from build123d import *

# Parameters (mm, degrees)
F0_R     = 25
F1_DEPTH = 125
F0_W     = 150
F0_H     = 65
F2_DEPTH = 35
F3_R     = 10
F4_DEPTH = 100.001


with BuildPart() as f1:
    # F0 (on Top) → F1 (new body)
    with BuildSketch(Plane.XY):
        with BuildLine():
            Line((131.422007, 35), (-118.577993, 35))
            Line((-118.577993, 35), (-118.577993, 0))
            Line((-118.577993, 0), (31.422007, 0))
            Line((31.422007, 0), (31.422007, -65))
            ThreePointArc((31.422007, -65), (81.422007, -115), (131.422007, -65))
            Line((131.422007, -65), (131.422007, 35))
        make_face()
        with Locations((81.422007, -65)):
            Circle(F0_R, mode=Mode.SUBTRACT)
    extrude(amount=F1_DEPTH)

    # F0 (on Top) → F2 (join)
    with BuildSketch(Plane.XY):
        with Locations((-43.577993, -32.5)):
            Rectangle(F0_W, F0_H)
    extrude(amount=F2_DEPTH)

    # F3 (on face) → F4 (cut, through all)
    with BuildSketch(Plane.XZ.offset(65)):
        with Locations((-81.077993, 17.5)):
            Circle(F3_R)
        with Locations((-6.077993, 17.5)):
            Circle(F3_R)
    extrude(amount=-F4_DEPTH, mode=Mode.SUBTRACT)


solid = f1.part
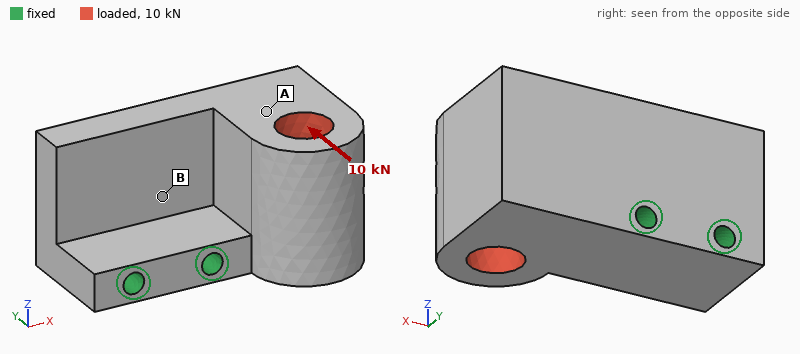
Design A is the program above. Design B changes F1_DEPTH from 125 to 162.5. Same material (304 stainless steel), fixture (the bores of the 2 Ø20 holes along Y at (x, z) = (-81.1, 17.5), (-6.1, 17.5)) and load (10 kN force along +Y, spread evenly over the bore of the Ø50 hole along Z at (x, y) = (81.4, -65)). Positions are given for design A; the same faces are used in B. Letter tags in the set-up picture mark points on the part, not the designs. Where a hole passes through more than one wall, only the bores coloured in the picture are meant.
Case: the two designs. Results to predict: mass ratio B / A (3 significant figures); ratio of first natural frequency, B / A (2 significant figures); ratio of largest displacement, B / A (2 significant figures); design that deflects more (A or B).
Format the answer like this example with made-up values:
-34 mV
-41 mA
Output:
1.27
0.78
1.4
B
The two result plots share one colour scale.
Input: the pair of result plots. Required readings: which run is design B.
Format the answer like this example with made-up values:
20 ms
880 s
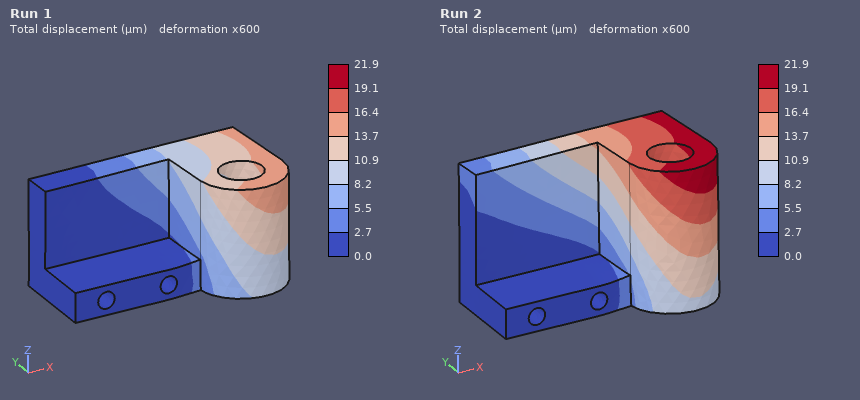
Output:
Run 2
